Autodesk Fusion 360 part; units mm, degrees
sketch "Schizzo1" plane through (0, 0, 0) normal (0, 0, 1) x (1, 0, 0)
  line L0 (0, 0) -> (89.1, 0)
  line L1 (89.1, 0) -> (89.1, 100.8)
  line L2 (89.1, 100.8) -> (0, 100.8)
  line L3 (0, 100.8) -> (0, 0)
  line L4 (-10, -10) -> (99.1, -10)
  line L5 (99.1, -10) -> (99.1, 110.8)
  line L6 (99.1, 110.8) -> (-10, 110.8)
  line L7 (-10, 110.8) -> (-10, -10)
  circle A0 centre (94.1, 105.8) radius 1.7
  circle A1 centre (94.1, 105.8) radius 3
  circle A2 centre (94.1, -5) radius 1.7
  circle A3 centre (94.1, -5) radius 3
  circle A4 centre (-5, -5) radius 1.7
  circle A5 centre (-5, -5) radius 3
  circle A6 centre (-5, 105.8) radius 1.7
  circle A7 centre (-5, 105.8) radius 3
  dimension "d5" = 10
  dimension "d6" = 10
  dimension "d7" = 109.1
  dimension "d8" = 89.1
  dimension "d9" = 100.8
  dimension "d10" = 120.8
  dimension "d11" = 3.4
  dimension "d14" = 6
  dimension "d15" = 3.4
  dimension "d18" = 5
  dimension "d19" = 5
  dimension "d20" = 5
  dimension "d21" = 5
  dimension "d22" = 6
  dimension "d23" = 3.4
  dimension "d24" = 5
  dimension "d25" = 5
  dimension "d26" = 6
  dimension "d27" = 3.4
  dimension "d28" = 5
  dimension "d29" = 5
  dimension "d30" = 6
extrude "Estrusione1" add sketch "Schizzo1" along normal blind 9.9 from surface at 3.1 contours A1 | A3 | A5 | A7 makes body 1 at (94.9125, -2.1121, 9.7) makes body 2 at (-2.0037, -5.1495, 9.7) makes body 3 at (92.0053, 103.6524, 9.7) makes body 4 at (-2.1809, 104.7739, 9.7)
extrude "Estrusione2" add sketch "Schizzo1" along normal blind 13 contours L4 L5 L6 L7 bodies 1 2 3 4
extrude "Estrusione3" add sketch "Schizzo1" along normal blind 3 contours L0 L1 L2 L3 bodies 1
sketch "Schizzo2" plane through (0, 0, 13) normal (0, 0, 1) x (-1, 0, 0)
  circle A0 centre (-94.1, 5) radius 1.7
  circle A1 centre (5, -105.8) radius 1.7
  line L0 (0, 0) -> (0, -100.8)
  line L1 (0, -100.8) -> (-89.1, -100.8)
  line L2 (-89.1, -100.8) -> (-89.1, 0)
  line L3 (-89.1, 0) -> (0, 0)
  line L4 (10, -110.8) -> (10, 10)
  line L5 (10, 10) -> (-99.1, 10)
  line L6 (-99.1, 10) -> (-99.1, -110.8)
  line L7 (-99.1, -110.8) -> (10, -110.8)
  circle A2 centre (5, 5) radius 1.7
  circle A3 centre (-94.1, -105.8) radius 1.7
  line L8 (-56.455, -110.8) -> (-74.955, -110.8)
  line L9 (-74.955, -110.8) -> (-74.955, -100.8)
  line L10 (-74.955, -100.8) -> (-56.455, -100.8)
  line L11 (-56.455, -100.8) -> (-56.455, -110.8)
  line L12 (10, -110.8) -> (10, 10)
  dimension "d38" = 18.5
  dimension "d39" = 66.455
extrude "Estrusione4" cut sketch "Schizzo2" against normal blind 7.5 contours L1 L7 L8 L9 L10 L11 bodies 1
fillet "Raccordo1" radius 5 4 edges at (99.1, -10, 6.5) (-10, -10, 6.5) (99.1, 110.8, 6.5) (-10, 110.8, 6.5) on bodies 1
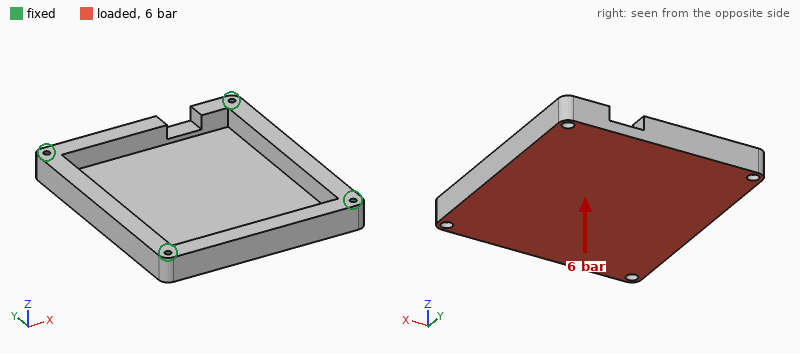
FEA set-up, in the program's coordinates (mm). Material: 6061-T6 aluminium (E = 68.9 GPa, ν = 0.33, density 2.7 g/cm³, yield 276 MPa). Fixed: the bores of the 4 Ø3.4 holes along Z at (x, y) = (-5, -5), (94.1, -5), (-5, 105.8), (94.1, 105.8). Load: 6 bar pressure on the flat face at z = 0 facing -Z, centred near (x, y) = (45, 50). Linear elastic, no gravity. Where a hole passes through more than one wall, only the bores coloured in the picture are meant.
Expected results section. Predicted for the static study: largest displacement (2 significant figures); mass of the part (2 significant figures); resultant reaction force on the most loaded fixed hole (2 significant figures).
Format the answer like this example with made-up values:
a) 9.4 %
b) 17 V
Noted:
a) 0.59 mm
b) 210 g
c) 3.3 kN
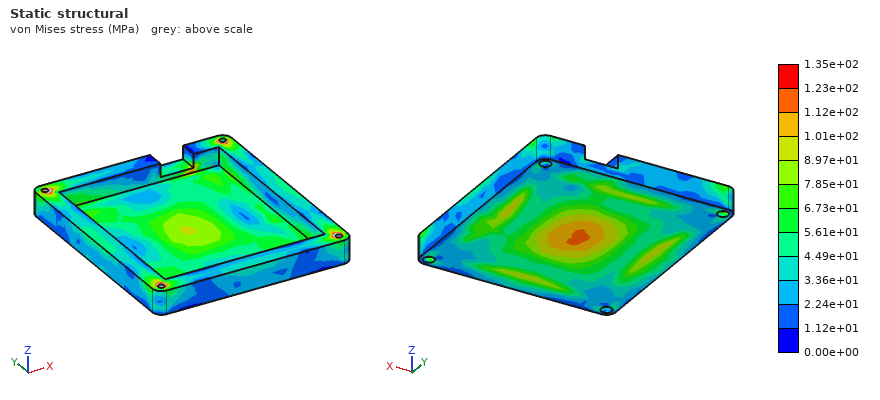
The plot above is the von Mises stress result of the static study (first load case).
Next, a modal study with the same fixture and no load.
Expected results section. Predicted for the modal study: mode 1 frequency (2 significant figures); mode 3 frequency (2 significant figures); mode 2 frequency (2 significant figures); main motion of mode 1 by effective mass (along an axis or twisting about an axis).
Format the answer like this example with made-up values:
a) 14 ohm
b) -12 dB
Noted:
a) 2300 Hz
b) 4000 Hz
c) 3900 Hz
d) along Z
